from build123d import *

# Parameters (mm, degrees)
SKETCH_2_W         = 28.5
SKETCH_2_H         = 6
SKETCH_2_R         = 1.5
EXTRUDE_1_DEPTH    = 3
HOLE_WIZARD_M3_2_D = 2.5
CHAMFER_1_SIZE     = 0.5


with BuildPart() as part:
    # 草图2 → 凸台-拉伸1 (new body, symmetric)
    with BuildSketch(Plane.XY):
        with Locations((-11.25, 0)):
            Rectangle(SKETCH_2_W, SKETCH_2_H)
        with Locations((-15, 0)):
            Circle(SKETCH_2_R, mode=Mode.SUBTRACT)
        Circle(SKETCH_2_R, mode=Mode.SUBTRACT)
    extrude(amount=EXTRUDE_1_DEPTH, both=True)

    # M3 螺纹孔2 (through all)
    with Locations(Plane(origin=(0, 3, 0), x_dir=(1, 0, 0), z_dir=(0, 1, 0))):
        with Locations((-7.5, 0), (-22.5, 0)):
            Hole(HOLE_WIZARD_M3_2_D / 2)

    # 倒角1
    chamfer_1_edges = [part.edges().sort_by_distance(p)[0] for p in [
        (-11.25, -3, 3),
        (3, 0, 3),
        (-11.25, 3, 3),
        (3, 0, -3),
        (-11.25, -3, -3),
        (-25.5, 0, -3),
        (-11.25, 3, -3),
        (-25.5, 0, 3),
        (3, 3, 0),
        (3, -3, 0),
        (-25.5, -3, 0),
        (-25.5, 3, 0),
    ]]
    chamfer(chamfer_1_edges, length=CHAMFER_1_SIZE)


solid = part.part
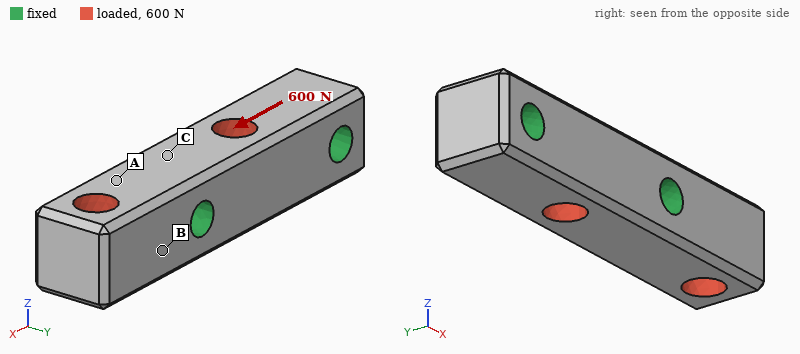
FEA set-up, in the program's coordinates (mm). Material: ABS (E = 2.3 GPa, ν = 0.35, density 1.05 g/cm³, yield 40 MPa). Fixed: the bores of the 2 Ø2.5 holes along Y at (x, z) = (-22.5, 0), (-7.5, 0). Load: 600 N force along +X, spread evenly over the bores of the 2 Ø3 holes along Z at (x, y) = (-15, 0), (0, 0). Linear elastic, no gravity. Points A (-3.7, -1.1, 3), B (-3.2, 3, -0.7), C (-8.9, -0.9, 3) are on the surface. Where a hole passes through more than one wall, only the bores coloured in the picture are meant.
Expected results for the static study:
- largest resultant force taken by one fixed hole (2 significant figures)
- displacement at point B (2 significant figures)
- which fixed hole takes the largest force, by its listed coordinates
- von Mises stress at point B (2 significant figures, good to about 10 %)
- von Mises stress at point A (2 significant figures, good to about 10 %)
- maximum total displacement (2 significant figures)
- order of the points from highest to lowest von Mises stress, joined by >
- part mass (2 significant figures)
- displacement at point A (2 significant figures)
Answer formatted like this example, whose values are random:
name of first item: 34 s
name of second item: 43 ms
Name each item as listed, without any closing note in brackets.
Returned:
largest resultant force taken by one fixed hole: 440 N
displacement at point B: 18 µm
which fixed hole takes the largest force, by its listed coordinates: (-7.5, 0)
von Mises stress at point B: 12 MPa
von Mises stress at point A: 6.3 MPa
maximum total displacement: 53 µm
order of the points from highest to lowest von Mises stress, joined by >: B > A > C
part mass: 0.91 g
displacement at point A: 14 µm
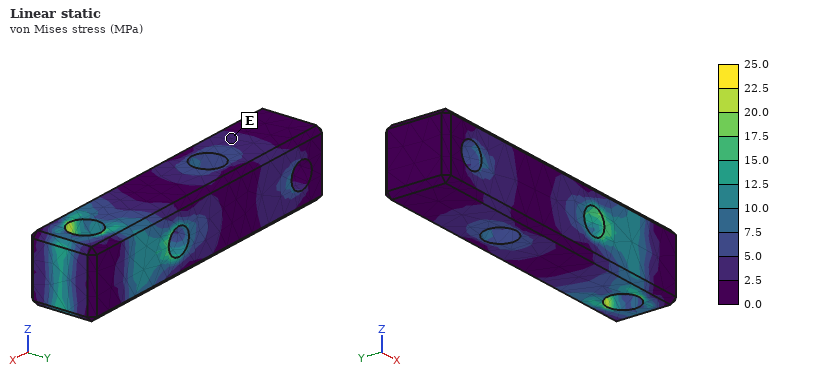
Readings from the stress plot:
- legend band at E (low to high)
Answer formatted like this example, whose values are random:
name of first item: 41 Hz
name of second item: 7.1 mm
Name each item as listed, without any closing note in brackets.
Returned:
legend band at E: 2.5 to 5.0 MPa
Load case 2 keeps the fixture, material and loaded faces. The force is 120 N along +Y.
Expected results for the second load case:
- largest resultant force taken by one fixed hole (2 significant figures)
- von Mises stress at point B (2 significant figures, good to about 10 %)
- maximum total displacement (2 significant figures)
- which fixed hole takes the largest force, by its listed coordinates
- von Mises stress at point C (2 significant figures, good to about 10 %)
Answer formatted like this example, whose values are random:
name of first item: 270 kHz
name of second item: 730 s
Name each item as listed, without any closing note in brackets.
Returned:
largest resultant force taken by one fixed hole: 91 N
von Mises stress at point B: 6.9 MPa
maximum total displacement: 79 µm
which fixed hole takes the largest force, by its listed coordinates: (-7.5, 0)
von Mises stress at point C: 2.1 MPa
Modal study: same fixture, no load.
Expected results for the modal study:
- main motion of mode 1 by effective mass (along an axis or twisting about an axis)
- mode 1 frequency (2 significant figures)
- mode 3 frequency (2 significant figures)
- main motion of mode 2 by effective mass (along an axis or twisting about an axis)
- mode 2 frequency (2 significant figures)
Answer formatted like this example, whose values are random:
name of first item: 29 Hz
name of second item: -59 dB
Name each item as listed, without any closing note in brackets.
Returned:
main motion of mode 1 by effective mass: along Z
mode 1 frequency: 10 kHz
mode 3 frequency: 21 kHz
main motion of mode 2 by effective mass: along Y
mode 2 frequency: 12 kHz
